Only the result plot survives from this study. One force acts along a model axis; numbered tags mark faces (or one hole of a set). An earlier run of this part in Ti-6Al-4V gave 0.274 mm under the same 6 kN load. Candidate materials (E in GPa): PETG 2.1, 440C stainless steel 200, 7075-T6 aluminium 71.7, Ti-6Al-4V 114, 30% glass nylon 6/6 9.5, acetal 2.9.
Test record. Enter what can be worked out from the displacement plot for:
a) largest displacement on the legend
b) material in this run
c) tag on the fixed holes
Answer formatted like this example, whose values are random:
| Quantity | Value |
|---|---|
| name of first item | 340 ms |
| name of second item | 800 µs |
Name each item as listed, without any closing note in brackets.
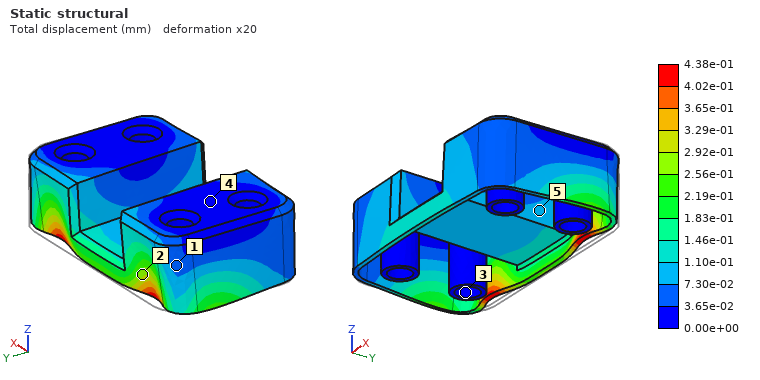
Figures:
| Quantity | Value |
|---|---|
| largest displacement on the legend | 4.38e-01 mm |
| material in this run | 7075-T6 aluminium |
| tag on the fixed holes | 3 |
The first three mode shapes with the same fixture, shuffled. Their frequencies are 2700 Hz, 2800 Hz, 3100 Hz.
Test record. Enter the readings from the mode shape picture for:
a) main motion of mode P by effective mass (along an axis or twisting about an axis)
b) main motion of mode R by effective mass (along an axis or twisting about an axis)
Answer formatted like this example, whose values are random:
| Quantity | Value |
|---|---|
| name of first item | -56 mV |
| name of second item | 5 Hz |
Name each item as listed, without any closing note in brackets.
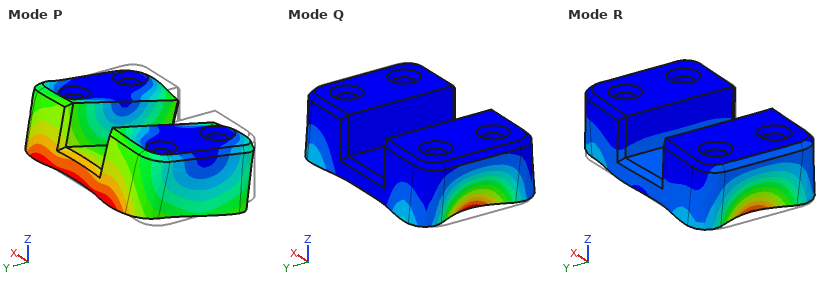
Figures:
| Quantity | Value |
|---|---|
| main motion of mode P by effective mass | along Y |
| main motion of mode R by effective mass | along X |
